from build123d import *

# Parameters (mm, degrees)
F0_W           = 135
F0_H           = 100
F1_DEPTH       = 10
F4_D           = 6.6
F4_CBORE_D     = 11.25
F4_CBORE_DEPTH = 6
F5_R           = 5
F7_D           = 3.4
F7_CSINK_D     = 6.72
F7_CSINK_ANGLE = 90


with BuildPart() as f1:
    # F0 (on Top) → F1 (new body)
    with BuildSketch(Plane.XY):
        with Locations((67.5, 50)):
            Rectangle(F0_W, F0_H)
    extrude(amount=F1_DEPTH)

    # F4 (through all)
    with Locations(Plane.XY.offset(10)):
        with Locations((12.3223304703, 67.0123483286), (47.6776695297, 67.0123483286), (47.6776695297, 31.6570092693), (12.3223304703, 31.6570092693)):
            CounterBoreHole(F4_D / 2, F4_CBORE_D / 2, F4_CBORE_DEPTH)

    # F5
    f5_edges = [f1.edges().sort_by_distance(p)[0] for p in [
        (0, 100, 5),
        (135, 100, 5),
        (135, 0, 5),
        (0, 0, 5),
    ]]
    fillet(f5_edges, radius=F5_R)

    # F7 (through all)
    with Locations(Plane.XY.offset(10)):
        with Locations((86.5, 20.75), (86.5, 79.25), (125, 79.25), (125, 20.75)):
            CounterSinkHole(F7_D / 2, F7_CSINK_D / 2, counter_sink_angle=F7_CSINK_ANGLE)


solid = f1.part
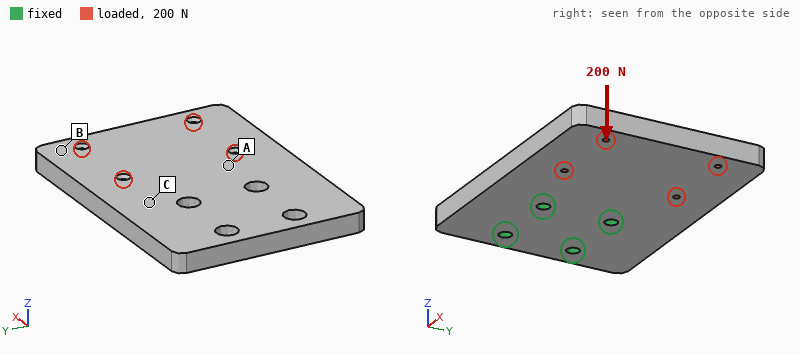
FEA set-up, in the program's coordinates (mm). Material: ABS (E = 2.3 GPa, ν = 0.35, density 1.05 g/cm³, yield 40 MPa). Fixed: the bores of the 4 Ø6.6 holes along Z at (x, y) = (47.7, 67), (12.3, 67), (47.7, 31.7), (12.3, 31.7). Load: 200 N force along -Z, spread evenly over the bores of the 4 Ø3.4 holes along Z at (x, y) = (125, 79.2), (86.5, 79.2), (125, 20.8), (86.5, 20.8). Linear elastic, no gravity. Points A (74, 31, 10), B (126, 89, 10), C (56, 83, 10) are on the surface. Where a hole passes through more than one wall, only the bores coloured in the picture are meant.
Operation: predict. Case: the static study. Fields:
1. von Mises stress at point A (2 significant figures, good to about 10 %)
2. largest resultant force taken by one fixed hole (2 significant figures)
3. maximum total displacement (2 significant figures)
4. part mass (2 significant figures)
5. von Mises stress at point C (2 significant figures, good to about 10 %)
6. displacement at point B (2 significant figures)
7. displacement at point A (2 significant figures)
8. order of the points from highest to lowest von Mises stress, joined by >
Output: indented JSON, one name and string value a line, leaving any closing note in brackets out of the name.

{
  "von Mises stress at point A": "3.2 MPa",
  "largest resultant force taken by one fixed hole": "310 N",
  "maximum total displacement": "1.7 mm",
  "part mass": "140 g",
  "von Mises stress at point C": "5.7 MPa",
  "displacement at point B": "1.5 mm",
  "displacement at point A": "0.36 mm",
  "order of the points from highest to lowest von Mises stress, joined by >": "C > A > B"
}
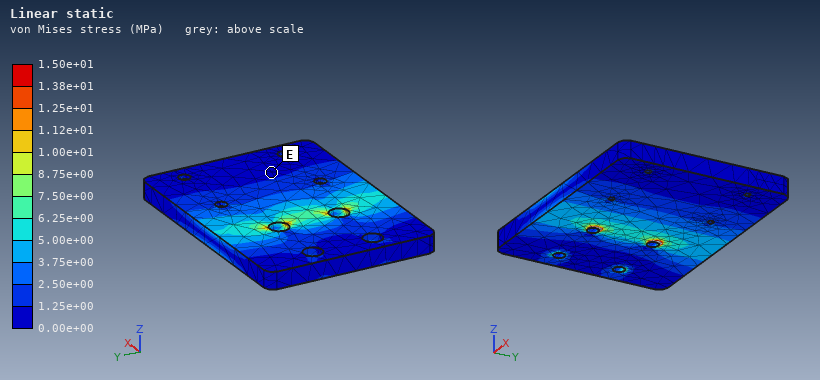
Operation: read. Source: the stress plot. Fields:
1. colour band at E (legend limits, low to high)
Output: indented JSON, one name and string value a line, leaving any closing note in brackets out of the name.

{
  "colour band at E": "0.00e+00 to 1.25e+00 MPa"
}
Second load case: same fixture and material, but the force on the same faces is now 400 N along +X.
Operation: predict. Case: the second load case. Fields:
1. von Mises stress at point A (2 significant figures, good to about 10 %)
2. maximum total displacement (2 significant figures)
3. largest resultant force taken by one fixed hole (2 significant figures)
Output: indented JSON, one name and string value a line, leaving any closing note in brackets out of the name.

{
  "von Mises stress at point A": "0.33 MPa",
  "maximum total displacement": "29 µm",
  "largest resultant force taken by one fixed hole": "140 N"
}
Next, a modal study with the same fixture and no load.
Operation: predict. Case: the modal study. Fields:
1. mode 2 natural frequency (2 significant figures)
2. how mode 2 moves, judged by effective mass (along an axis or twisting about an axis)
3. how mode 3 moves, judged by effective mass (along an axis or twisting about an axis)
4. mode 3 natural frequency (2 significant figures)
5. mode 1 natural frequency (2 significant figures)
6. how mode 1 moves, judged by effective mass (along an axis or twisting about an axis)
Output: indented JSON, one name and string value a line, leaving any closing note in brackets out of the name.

{
  "mode 2 natural frequency": "540 Hz",
  "how mode 2 moves, judged by effective mass": "twisting about X",
  "how mode 3 moves, judged by effective mass": "along Y",
  "mode 3 natural frequency": "1200 Hz",
  "mode 1 natural frequency": "260 Hz",
  "how mode 1 moves, judged by effective mass": "along Z"
}
